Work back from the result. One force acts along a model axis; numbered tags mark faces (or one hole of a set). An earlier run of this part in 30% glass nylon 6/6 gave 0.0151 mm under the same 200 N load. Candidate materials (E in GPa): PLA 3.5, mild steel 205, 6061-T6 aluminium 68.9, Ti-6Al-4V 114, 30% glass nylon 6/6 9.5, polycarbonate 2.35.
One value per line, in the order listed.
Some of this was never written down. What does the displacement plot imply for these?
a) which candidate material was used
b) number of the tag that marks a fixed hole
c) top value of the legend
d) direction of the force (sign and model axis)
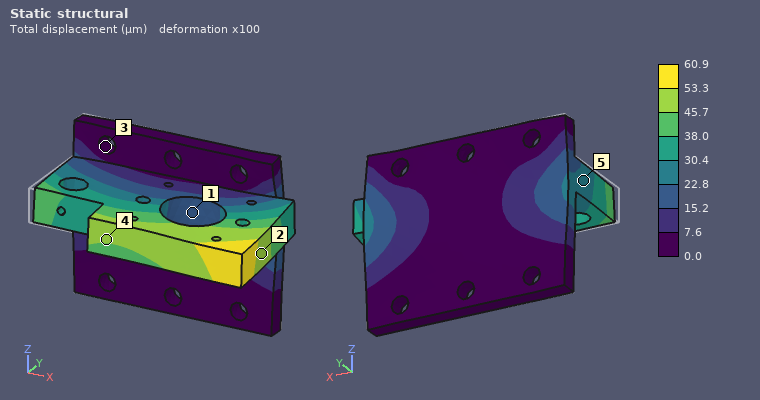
polycarbonate
3
60.9 µm
+X
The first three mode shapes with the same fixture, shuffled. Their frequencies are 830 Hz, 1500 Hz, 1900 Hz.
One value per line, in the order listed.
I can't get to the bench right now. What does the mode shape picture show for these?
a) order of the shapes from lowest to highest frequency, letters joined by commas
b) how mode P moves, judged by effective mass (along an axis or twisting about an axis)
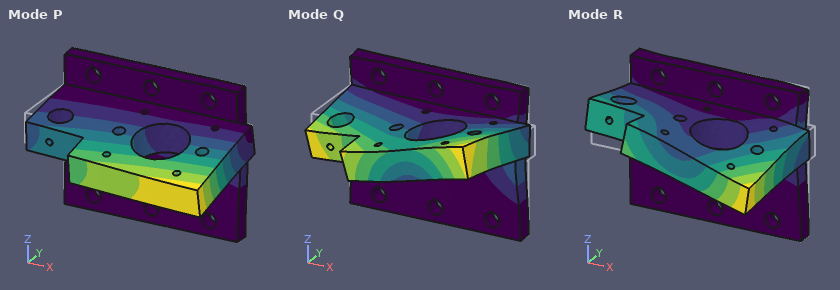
P, Q, R
along Z
